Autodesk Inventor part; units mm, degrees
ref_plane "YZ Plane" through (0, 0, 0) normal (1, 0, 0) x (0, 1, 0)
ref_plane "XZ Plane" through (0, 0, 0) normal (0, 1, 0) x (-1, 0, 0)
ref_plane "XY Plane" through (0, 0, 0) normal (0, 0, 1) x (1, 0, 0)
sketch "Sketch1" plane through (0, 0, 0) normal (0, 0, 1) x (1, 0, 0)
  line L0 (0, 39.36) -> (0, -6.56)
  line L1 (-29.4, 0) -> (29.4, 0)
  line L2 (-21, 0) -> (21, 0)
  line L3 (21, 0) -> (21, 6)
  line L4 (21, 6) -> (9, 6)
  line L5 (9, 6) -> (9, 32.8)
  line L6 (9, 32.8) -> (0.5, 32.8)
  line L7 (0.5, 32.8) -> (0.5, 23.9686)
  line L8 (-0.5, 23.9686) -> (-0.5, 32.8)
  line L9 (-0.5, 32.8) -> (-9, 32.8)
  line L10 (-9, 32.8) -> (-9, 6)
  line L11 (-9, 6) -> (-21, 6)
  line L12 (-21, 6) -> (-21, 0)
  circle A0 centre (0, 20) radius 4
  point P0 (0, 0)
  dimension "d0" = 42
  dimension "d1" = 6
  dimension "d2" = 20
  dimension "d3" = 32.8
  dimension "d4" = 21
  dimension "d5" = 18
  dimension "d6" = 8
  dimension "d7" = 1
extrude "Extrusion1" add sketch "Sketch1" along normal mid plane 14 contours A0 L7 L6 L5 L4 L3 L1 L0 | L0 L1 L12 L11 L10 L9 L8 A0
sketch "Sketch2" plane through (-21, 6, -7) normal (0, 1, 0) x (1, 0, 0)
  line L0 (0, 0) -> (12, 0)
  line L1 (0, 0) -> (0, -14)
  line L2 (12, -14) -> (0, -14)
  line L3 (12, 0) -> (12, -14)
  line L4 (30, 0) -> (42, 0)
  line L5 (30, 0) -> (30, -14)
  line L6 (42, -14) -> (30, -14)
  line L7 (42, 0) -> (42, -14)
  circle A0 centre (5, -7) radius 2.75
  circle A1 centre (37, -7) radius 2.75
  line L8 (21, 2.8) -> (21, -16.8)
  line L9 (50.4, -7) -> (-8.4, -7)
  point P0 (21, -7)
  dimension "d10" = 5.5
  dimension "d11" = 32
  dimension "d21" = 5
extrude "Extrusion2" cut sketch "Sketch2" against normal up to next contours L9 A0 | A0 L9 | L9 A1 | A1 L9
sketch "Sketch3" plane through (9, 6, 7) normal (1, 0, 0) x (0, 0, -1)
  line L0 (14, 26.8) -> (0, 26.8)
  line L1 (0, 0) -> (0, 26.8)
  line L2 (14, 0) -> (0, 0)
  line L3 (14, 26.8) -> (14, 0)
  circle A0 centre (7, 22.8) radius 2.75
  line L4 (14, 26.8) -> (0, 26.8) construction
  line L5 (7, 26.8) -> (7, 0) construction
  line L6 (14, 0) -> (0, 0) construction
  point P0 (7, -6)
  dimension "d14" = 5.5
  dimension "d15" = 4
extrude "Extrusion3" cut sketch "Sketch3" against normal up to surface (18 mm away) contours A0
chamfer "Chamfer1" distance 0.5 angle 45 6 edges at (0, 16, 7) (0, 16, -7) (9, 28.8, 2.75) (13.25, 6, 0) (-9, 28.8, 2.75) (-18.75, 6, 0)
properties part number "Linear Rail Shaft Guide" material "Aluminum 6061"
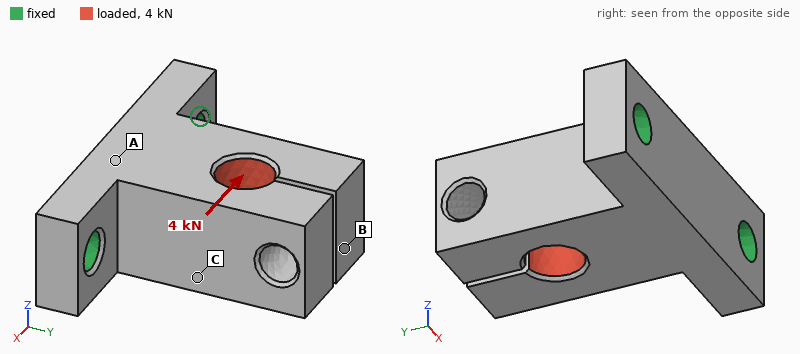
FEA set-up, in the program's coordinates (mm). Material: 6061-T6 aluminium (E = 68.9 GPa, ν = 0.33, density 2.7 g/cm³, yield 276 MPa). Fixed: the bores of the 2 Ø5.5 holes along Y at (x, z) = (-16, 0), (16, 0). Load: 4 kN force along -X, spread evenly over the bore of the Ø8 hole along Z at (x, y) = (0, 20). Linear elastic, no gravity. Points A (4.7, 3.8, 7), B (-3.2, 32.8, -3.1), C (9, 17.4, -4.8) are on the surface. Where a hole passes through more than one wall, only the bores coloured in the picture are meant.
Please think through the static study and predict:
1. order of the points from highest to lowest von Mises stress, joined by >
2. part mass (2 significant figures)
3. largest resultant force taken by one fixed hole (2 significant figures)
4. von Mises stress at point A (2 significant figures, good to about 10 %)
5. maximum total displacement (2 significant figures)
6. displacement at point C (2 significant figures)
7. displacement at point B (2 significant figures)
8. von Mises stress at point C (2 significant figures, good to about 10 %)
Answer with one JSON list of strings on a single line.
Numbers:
["C > A > B", "24 g", "3.4 kN", "30 MPa", "0.12 mm", "0.047 mm", "0.12 mm", "58 MPa"]
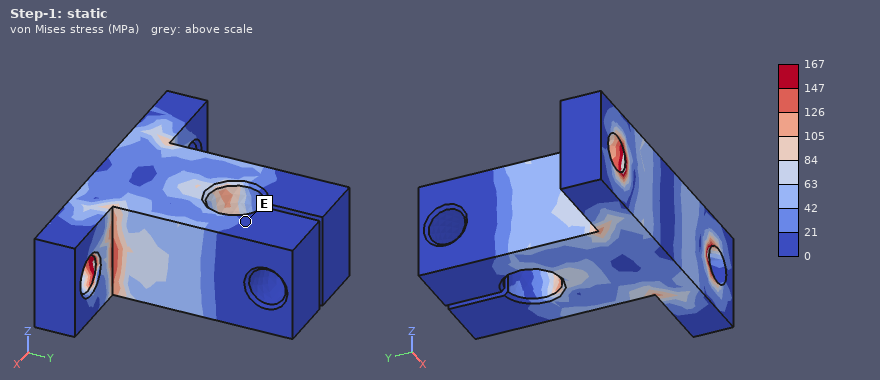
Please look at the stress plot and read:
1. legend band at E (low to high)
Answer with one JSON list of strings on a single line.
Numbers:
["0 to 21 MPa"]
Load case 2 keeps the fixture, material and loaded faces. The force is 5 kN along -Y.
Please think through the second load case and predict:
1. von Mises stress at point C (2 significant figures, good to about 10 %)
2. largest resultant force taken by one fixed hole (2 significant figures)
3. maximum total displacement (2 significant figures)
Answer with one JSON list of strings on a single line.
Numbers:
["45 MPa", "2.7 kN", "67 µm"]
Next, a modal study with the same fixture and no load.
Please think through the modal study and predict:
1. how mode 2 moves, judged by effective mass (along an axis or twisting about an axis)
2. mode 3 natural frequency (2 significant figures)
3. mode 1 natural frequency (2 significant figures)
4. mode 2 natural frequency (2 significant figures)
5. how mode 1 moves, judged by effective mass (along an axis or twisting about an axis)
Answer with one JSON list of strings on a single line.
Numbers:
["along X", "11 kHz", "5200 Hz", "8600 Hz", "along Z"]
